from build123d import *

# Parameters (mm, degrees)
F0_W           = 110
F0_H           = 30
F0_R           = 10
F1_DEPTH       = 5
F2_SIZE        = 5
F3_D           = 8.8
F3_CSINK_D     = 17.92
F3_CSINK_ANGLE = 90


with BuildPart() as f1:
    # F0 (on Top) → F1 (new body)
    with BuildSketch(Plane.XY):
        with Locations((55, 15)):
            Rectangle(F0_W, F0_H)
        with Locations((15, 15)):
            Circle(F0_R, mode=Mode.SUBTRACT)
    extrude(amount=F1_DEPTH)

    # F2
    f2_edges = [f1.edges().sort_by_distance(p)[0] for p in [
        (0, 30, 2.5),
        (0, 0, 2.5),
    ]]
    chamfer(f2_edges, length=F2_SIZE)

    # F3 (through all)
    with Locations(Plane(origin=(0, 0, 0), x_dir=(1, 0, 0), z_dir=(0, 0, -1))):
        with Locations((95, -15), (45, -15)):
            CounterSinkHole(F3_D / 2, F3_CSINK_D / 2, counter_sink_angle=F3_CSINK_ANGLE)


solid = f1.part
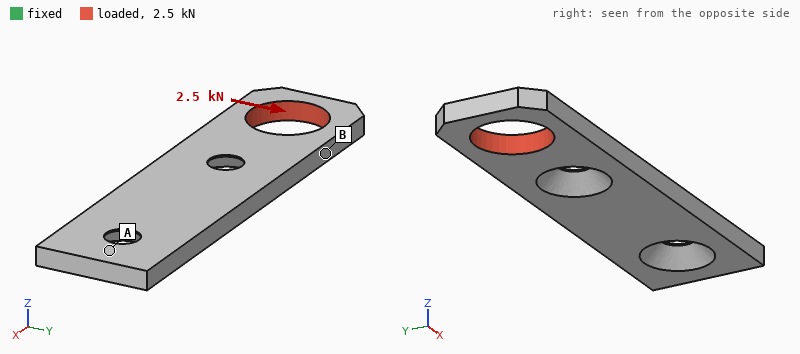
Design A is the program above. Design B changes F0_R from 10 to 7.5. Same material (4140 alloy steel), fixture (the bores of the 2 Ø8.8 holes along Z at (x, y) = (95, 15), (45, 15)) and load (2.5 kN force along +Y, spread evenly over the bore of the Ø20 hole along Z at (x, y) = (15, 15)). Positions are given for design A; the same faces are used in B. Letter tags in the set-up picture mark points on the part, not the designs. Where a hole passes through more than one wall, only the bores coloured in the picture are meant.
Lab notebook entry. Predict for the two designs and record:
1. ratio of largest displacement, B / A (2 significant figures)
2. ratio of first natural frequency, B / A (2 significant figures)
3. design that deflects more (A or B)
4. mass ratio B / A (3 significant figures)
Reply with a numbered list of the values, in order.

1. 0.81
2. 0.93
3. A
4. 1.05
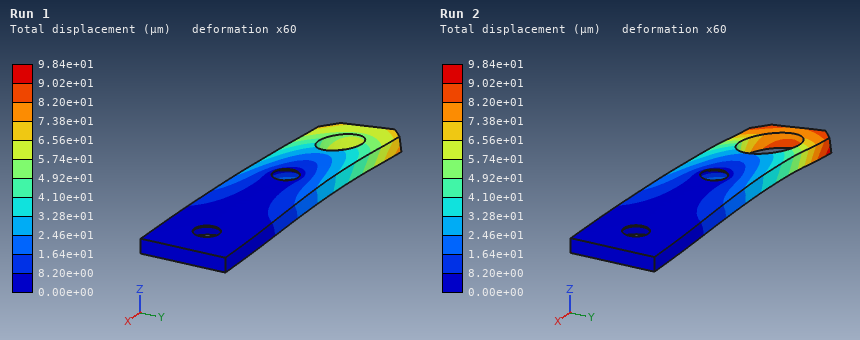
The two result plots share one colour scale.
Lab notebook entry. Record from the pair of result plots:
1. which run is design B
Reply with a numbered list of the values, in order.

1. Run 1
